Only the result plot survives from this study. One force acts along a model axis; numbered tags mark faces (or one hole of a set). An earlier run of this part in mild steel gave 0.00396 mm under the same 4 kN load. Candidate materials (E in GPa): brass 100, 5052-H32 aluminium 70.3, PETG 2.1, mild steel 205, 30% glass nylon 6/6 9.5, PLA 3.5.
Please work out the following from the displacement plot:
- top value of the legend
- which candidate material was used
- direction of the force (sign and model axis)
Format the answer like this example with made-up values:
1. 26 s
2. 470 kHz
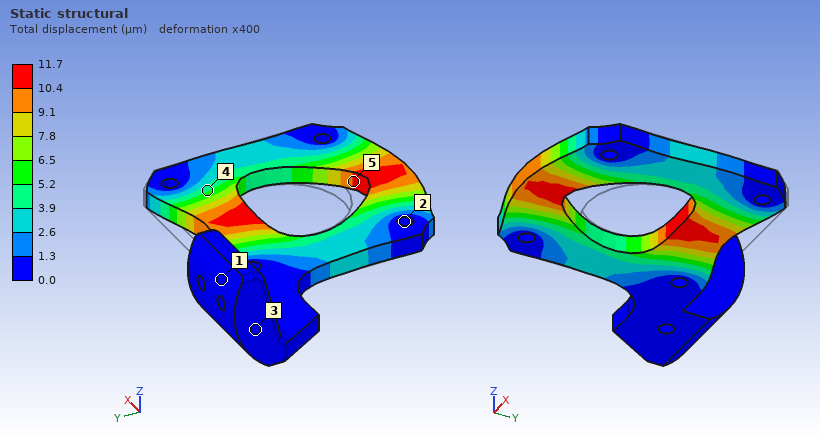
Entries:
1. 11.7 µm
2. 5052-H32 aluminium
3. -Y
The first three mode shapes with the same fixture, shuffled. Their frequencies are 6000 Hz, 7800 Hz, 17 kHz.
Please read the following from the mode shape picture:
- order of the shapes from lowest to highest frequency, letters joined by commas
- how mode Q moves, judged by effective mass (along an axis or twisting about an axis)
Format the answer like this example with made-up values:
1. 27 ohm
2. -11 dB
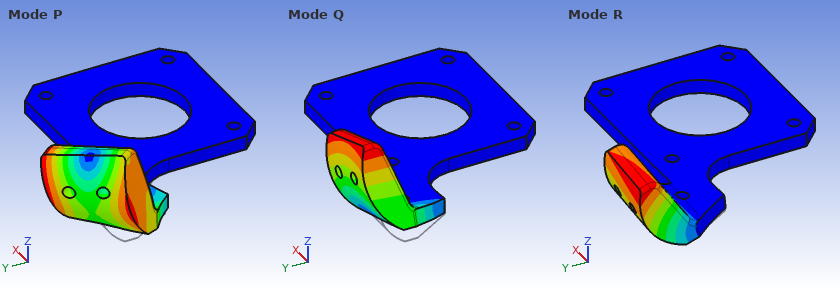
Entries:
1. R, Q, P
2. along X
